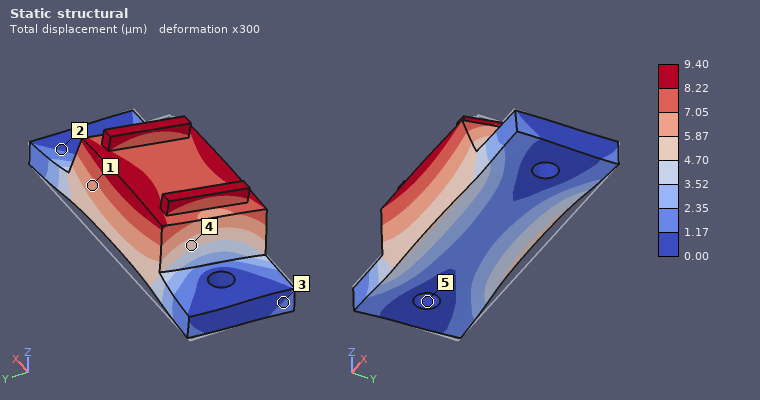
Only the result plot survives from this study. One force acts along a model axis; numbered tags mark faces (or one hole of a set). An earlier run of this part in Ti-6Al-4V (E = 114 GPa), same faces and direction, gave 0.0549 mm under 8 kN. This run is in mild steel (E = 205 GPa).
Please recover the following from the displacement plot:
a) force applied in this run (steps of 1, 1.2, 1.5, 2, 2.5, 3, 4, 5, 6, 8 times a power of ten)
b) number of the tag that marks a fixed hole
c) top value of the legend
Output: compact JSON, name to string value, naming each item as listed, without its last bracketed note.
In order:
{"force applied in this run": "2.5 kN", "number of the tag that marks a fixed hole": "5", "top value of the legend": "9.40 µm"}
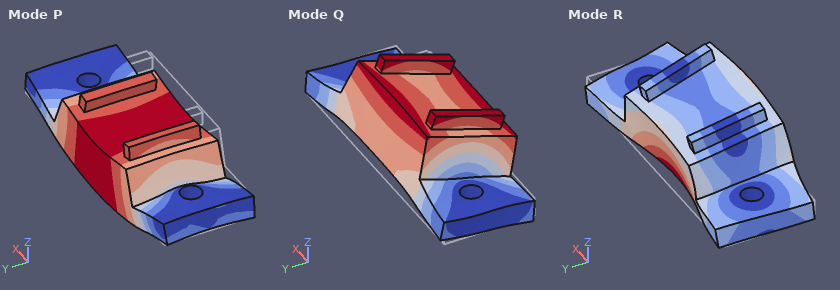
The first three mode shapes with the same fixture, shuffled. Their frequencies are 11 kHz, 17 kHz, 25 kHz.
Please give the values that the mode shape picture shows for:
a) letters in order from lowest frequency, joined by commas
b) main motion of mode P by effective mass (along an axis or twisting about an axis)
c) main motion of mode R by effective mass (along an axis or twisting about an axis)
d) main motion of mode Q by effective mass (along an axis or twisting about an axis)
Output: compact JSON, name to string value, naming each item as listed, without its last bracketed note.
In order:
{"letters in order from lowest frequency, joined by commas": "Q, P, R", "main motion of mode P by effective mass": "along Z", "main motion of mode R by effective mass": "along Y", "main motion of mode Q by effective mass": "along Y"}
